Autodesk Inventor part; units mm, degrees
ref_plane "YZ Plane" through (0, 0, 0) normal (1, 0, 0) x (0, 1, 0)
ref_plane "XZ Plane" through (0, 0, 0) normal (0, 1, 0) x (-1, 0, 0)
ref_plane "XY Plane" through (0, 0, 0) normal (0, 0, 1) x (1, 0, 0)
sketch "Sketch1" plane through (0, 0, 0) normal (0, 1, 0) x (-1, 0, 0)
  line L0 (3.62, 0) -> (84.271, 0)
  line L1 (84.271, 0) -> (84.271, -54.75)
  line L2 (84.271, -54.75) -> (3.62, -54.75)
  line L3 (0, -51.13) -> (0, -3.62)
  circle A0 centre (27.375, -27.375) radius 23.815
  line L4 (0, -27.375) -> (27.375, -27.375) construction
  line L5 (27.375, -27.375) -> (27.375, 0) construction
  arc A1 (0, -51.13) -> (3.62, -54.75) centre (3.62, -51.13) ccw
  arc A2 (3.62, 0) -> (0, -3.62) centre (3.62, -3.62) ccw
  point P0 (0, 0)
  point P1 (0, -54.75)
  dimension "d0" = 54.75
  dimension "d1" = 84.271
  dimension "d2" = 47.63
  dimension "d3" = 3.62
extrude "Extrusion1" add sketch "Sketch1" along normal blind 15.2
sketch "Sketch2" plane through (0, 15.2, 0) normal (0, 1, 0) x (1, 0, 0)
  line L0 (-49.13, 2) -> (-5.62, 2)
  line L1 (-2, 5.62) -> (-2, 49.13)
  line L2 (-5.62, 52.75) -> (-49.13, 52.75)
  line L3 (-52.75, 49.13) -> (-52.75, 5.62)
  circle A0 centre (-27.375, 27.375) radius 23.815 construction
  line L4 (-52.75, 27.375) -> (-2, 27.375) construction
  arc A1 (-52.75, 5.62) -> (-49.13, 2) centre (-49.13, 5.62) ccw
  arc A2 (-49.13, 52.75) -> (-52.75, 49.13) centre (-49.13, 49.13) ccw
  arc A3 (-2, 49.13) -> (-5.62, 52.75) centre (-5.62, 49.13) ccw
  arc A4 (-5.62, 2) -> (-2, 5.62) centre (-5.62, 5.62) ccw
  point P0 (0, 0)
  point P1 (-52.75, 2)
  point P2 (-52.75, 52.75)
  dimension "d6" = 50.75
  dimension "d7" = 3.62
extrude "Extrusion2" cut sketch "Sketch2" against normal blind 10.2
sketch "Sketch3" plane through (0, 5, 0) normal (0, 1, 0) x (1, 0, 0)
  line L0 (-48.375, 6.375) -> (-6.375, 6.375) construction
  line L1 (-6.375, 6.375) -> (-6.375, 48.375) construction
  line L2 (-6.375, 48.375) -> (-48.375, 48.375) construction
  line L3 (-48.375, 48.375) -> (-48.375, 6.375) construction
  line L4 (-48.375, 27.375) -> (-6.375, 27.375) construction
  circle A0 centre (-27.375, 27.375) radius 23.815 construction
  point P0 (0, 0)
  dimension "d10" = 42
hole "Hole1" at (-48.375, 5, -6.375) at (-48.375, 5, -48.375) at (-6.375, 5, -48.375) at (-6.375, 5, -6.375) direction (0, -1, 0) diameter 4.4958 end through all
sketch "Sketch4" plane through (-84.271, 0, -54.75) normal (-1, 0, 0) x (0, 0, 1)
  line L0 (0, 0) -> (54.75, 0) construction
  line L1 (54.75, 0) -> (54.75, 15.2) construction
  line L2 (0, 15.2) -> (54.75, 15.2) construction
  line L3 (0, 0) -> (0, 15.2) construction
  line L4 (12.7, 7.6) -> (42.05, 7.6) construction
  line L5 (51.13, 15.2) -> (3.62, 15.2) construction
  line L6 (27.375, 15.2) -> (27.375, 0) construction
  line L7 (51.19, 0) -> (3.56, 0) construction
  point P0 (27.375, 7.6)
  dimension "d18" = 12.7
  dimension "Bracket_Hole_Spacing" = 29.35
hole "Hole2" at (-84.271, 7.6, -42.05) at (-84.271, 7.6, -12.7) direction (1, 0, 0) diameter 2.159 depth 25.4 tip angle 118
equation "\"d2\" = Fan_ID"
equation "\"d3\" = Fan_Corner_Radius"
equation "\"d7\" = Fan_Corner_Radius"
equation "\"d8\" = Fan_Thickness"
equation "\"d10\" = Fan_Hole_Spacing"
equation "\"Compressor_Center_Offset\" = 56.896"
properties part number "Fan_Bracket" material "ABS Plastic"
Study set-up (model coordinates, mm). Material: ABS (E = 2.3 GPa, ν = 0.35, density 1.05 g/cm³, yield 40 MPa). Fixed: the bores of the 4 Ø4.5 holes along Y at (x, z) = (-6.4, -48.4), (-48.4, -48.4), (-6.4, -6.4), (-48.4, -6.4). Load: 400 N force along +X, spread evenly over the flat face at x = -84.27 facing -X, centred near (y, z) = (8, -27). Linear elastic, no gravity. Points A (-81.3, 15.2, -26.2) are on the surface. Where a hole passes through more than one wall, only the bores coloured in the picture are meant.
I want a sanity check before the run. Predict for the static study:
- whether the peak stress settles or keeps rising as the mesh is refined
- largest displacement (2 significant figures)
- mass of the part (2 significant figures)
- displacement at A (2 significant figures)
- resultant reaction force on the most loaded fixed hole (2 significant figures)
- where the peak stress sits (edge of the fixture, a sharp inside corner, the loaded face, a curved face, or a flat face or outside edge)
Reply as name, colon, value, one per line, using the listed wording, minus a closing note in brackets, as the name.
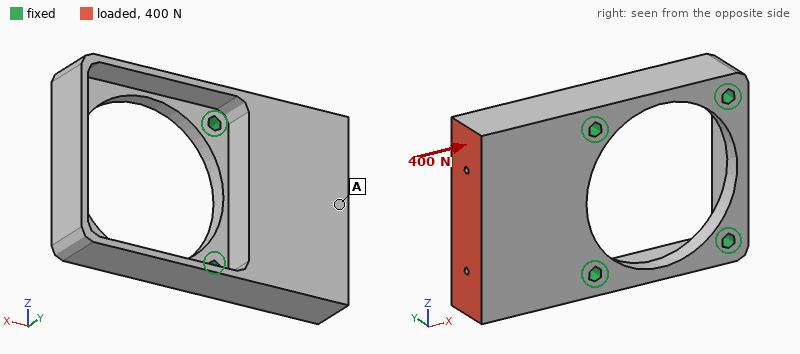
whether the peak stress settles or keeps rising as the mesh is refined: keeps rising
largest displacement: 0.18 mm
mass of the part: 36 g
displacement at A: 0.17 mm
resultant reaction force on the most loaded fixed hole: 180 N
where the peak stress sits: edge of the fixture
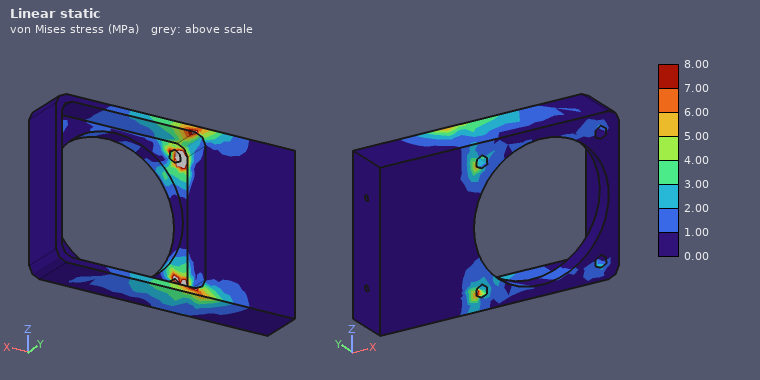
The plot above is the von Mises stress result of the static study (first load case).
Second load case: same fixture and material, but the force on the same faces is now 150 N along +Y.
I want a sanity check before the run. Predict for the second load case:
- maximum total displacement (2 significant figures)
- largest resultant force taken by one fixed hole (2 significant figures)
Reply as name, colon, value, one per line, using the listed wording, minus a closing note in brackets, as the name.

maximum total displacement: 0.54 mm
largest resultant force taken by one fixed hole: 130 N
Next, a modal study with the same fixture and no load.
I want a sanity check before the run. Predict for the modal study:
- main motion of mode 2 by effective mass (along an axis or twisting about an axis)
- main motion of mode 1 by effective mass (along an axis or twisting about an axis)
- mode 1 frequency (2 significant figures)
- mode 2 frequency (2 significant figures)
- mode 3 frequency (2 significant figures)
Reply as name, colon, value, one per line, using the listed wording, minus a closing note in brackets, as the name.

main motion of mode 2 by effective mass: twisting about X
main motion of mode 1 by effective mass: along Y
mode 1 frequency: 850 Hz
mode 2 frequency: 2700 Hz
mode 3 frequency: 3200 Hz
